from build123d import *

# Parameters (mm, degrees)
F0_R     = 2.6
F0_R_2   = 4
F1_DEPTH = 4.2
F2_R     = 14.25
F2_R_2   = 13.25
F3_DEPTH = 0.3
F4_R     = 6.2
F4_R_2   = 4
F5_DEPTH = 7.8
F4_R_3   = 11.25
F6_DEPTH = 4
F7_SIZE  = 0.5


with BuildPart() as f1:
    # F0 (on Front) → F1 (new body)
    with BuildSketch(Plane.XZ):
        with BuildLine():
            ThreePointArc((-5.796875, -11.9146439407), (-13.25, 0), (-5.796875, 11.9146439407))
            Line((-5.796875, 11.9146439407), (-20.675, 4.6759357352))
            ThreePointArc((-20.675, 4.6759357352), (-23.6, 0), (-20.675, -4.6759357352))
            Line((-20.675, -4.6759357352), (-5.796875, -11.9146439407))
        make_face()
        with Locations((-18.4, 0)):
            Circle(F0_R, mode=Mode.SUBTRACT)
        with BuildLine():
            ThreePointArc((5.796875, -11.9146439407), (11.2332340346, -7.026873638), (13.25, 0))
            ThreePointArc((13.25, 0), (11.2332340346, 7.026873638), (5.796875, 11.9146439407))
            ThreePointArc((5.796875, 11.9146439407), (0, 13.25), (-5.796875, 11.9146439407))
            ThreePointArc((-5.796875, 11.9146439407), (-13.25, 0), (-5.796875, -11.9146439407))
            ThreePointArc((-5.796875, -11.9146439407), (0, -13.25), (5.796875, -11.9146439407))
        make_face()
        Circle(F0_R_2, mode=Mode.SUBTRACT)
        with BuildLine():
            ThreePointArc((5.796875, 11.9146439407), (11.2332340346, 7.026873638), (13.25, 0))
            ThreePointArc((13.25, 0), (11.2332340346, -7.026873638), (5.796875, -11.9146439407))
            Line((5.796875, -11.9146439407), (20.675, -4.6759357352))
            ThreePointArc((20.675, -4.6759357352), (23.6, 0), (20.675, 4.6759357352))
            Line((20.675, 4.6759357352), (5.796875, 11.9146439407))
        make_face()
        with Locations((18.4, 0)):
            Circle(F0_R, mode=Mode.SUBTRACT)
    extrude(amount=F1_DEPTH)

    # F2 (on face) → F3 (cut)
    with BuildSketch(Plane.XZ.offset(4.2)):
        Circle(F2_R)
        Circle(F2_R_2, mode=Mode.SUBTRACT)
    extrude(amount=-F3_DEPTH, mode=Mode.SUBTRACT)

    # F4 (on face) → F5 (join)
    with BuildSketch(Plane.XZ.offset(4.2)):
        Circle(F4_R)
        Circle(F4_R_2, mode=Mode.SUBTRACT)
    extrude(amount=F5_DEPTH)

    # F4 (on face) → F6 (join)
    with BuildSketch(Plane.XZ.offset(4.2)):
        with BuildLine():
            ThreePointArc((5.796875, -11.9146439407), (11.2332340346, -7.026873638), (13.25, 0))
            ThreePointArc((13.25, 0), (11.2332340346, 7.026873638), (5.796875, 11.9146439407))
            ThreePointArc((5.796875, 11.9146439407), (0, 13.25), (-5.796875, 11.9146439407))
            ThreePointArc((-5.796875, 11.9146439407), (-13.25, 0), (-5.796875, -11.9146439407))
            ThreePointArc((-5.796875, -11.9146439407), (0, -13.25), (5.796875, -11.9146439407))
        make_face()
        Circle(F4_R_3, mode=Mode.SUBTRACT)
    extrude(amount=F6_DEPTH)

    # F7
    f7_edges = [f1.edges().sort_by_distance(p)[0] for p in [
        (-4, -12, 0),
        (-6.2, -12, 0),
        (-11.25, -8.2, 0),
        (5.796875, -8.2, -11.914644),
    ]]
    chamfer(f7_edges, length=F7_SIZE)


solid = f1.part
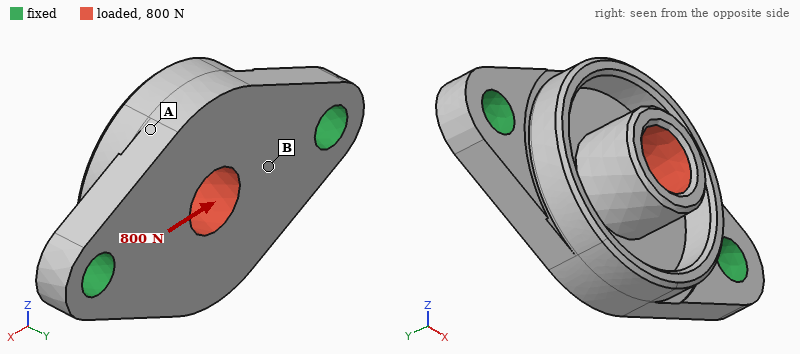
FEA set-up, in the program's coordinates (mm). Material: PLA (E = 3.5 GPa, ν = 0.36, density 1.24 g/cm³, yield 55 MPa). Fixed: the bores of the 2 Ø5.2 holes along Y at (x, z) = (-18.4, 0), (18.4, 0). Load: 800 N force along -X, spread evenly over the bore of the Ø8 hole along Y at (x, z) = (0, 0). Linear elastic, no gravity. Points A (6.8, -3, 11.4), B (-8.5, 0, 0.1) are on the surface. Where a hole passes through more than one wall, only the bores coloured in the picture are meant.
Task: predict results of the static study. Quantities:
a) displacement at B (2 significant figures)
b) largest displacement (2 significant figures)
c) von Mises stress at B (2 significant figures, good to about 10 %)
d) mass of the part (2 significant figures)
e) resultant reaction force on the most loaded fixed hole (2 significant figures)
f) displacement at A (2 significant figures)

0.041 mm
0.15 mm
7.5 MPa
5.2 g
420 N
0.029 mm
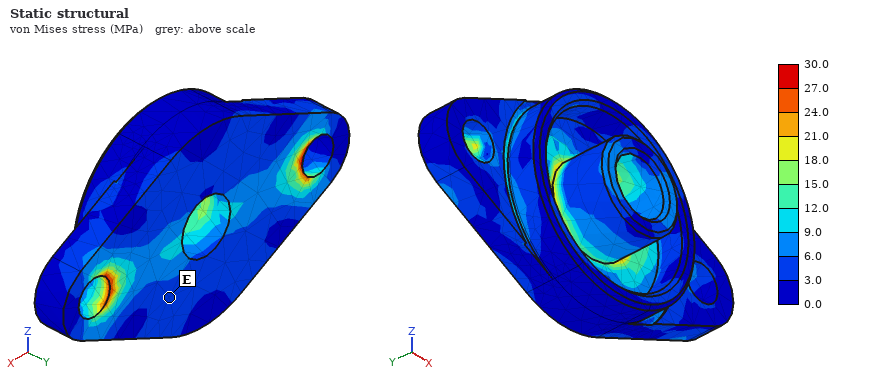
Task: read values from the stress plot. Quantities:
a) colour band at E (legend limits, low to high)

3.0 to 6.0 MPa
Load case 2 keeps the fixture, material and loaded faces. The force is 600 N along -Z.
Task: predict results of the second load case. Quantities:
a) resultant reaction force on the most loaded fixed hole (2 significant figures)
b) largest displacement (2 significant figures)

300 N
0.33 mm
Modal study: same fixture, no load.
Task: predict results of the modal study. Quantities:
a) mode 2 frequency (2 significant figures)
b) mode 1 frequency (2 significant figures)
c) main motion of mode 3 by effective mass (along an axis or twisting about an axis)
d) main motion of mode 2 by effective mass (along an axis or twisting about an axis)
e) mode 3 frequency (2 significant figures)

4400 Hz
3600 Hz
along Z
along Y
9200 Hz
